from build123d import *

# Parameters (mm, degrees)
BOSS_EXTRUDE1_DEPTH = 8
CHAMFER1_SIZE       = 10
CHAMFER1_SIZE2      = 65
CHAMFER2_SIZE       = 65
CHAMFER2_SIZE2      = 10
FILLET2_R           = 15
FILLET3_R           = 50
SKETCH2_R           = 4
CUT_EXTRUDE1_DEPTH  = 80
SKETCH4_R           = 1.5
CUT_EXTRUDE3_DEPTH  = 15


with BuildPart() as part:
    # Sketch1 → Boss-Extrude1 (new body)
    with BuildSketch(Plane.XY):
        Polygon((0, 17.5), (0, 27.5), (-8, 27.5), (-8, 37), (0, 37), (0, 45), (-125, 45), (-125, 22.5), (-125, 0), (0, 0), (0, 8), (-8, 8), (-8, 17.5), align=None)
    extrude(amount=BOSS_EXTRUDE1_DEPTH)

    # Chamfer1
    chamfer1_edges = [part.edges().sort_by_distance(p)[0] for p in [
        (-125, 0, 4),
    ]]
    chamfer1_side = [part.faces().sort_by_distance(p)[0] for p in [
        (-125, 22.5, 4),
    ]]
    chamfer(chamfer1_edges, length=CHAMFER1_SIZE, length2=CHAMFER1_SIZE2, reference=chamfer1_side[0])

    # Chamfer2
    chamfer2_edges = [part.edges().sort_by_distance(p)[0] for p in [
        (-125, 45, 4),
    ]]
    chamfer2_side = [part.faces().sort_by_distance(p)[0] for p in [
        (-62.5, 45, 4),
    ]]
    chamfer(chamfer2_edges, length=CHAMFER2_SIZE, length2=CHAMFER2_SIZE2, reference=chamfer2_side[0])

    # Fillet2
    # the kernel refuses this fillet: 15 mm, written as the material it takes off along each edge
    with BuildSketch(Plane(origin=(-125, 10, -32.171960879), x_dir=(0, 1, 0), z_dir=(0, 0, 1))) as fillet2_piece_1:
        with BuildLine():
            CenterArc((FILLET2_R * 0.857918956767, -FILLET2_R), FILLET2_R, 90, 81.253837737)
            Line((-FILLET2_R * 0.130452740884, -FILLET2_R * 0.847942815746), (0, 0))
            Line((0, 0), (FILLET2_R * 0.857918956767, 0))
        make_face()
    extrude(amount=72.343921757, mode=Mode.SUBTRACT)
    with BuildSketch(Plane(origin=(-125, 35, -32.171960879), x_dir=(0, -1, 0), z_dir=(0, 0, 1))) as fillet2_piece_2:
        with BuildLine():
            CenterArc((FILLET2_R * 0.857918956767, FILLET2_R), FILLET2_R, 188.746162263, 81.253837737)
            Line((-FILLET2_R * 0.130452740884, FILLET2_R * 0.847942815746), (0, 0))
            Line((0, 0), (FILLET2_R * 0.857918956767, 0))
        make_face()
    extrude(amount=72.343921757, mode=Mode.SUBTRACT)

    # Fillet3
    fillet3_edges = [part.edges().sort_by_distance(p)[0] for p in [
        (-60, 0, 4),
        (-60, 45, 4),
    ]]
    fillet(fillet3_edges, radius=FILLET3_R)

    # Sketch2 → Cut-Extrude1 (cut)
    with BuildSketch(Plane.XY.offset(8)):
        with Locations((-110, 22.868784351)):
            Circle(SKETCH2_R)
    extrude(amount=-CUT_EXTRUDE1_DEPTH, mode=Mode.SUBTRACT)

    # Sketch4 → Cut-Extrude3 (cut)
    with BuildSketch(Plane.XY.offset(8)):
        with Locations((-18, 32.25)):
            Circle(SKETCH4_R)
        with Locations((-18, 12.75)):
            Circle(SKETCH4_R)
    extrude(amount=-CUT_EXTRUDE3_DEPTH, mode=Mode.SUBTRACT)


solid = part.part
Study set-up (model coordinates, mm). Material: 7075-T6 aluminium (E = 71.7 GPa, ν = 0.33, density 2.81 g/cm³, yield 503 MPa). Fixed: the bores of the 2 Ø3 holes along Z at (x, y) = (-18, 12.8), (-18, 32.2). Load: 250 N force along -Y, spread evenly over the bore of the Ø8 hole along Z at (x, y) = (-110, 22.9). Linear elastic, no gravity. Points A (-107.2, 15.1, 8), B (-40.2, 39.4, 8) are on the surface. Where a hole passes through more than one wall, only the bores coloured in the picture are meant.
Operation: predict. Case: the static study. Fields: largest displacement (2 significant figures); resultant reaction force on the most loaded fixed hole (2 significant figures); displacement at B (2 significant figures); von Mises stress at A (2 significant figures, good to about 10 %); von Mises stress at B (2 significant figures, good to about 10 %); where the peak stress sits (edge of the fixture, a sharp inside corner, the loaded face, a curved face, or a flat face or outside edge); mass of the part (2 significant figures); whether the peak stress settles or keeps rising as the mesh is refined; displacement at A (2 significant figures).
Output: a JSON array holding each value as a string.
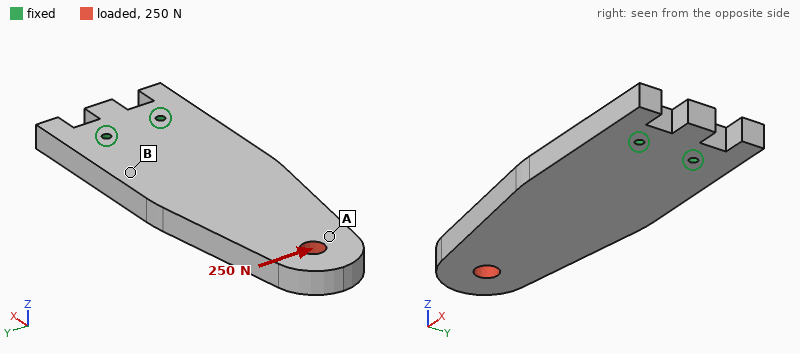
["34 µm", "1.1 kN", "5.8 µm", "2.1 MPa", "4.8 MPa", "edge of the fixture", "110 g", "keeps rising", "28 µm"]
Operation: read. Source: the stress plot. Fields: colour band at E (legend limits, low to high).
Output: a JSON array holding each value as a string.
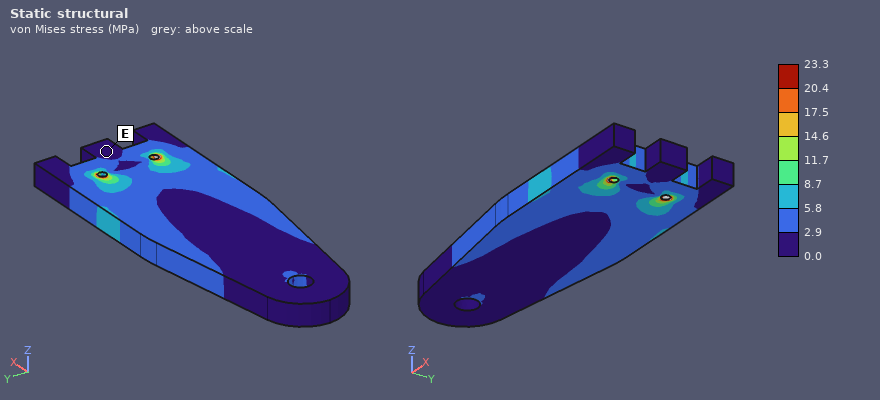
["0.0 to 2.9 MPa"]
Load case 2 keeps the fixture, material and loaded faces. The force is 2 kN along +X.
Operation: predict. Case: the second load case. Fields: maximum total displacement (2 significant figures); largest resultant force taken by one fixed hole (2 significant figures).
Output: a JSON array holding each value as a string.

["11 µm", "1.0 kN"]
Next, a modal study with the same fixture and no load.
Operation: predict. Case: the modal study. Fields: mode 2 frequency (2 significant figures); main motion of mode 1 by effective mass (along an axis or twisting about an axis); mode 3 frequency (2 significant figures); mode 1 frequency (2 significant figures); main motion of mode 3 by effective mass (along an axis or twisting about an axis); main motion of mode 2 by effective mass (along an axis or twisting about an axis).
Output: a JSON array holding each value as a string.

["2700 Hz", "along Z", "3600 Hz", "680 Hz", "twisting about X", "along Y"]
